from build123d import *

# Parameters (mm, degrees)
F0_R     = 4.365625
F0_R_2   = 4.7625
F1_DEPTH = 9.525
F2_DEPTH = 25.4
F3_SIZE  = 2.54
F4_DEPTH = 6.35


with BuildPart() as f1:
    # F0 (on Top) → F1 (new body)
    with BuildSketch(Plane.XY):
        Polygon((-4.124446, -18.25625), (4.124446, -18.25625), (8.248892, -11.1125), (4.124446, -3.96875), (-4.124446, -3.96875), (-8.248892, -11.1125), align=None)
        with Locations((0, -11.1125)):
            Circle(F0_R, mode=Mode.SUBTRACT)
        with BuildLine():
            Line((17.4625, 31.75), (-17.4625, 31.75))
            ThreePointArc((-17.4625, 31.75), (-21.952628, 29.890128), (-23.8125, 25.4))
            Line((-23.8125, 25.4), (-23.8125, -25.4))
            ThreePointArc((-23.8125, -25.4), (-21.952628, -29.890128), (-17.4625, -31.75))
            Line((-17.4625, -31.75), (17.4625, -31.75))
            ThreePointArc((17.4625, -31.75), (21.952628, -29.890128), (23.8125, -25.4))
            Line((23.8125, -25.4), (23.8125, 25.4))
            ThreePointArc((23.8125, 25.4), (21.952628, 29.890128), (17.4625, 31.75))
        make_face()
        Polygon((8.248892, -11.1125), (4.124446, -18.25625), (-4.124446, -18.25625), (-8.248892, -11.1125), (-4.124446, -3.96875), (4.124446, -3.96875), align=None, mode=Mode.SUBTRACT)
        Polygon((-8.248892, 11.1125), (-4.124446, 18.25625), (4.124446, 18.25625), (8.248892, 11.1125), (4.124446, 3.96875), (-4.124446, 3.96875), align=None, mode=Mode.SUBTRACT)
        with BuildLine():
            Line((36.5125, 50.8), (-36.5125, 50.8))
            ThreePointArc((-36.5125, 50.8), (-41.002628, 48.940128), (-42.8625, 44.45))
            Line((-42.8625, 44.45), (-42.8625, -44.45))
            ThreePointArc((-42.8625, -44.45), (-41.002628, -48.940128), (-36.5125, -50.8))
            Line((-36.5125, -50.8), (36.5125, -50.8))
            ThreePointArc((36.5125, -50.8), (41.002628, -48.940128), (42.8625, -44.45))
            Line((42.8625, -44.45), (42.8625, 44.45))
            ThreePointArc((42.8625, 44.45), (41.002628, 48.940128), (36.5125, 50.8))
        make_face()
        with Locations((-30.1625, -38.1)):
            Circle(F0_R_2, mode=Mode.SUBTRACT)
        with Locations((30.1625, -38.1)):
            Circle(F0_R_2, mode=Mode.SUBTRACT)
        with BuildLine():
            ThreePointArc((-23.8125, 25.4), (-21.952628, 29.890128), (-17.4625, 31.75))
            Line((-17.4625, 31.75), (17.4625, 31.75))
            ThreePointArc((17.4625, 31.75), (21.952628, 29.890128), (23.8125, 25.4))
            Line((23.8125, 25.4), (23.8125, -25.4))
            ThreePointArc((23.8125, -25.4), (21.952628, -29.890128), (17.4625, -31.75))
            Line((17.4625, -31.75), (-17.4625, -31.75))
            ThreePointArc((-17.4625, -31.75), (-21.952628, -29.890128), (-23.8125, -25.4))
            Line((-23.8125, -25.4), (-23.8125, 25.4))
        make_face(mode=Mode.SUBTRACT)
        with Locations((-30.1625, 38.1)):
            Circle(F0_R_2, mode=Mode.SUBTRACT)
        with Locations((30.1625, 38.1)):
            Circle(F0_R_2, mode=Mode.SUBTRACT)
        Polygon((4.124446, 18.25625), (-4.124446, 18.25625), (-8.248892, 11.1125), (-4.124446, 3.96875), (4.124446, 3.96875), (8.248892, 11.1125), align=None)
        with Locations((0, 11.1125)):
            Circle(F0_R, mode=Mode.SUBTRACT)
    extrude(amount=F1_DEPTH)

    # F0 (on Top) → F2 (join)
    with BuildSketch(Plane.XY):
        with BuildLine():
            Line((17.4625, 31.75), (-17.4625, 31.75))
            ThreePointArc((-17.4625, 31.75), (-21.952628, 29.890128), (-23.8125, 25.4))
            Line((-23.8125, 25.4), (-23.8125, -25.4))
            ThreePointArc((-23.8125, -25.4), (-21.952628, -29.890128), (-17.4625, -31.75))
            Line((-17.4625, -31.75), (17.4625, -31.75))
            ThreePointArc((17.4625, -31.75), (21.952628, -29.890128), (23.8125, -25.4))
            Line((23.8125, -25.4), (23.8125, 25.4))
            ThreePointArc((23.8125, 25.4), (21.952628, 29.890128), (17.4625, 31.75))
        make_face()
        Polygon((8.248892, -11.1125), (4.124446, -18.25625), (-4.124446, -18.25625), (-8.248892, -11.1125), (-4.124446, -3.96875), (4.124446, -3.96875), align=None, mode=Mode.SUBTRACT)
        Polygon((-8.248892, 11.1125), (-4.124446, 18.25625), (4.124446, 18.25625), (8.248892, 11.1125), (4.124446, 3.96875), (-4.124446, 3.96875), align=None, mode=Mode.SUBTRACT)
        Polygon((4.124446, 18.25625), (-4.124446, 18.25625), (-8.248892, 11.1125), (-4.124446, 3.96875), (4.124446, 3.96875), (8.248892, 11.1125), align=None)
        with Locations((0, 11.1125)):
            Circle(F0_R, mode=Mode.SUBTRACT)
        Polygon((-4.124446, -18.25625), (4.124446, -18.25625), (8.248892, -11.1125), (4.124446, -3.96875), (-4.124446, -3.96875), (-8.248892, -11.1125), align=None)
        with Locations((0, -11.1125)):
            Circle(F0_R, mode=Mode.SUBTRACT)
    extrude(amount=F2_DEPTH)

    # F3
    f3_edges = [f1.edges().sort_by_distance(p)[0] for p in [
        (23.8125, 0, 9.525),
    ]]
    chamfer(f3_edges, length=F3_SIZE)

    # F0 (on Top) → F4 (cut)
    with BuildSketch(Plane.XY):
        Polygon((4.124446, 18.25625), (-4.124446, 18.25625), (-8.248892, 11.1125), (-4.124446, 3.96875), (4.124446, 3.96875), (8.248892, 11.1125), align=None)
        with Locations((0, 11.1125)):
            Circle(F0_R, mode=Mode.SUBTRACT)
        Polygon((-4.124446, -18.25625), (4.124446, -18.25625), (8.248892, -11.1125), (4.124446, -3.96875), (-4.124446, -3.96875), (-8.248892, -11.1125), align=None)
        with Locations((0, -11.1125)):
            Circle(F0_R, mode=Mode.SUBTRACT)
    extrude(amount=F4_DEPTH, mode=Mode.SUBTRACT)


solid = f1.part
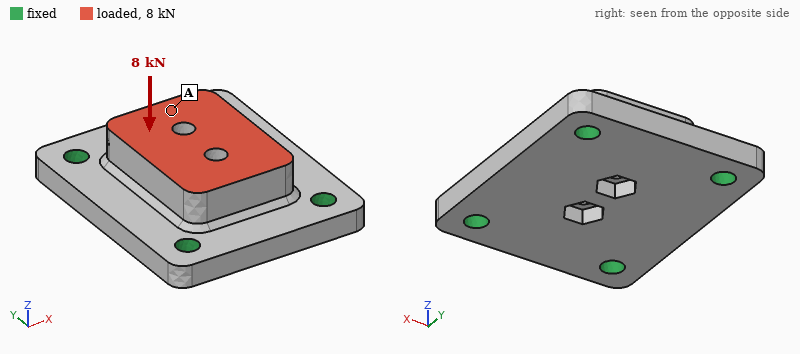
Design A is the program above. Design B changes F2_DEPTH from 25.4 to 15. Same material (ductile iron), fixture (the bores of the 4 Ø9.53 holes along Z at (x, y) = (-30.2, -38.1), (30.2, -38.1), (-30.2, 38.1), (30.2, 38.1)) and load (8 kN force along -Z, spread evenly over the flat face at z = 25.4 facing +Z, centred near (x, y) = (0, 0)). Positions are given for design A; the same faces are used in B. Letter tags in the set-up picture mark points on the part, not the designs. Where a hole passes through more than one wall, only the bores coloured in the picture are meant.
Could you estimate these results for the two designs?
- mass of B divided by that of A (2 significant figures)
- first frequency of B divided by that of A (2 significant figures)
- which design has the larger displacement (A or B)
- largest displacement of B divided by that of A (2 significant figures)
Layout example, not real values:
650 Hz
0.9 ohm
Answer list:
0.76
0.94
B
2.2
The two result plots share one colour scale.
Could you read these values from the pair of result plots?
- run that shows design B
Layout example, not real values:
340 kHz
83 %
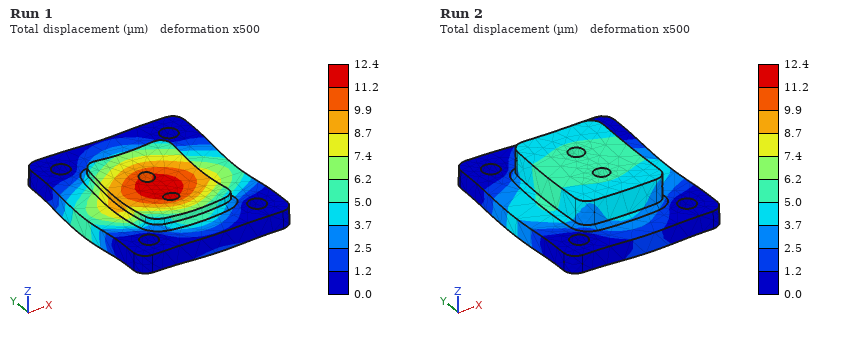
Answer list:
Run 1
